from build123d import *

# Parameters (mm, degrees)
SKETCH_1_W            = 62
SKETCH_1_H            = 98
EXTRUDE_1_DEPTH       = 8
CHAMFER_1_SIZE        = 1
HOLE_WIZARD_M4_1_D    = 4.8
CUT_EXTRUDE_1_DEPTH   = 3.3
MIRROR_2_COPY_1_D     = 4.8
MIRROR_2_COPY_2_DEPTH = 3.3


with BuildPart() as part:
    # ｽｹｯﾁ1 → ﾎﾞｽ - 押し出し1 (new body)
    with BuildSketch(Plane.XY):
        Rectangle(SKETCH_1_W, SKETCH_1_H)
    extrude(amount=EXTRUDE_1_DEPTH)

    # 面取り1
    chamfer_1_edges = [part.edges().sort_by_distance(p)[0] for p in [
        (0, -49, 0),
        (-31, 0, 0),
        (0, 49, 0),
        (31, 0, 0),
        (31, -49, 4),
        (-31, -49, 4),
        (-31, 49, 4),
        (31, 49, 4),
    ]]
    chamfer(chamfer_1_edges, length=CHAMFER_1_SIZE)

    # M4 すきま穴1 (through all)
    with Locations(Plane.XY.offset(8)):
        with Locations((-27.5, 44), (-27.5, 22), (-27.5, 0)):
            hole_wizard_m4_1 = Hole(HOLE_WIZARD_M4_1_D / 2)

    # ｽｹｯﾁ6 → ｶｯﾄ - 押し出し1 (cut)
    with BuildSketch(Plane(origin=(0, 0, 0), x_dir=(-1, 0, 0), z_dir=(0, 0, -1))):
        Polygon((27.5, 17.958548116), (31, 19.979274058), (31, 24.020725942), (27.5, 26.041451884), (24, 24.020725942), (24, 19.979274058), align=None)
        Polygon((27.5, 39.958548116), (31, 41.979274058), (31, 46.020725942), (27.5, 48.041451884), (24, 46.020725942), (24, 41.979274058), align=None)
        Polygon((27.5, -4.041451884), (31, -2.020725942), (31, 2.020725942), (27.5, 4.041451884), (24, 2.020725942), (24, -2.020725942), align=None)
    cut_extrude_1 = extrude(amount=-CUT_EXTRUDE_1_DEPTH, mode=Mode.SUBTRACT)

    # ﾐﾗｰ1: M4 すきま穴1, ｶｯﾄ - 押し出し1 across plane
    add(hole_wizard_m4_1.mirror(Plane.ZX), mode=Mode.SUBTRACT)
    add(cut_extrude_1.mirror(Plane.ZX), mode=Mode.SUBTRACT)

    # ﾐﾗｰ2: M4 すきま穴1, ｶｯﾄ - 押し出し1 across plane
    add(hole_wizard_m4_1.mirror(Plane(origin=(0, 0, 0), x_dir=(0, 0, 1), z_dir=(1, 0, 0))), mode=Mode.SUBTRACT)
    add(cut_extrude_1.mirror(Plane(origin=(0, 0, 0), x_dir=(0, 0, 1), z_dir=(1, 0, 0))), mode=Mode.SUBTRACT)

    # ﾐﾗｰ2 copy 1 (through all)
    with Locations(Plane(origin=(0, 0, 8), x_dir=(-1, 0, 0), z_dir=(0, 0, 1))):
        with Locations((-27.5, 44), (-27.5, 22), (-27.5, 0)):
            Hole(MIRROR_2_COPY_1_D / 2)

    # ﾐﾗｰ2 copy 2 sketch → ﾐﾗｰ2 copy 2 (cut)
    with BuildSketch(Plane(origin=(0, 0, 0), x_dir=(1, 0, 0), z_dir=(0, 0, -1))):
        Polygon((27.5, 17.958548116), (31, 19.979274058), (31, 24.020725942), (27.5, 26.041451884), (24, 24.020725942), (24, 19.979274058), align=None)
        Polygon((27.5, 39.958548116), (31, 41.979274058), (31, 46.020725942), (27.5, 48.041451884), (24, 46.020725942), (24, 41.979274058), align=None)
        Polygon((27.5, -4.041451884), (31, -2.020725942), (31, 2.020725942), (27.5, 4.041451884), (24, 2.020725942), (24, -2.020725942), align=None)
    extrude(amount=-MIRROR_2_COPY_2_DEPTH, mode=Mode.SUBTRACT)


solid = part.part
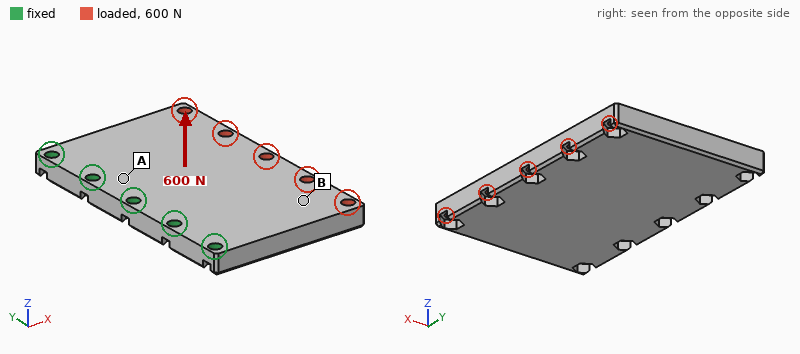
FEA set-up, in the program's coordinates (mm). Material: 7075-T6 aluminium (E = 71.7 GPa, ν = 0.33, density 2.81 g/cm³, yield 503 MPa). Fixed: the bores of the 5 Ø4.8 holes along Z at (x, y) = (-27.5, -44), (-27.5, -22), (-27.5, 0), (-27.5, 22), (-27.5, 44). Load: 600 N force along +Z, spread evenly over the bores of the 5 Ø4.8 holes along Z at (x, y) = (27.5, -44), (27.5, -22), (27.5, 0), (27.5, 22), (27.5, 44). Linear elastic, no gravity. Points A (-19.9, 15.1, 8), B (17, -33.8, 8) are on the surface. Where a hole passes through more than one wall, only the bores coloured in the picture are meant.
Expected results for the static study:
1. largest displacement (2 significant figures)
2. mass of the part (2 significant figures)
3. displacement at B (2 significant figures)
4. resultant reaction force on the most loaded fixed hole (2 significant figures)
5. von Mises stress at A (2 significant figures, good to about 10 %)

0.19 mm
130 g
0.13 mm
200 N
24 MPa
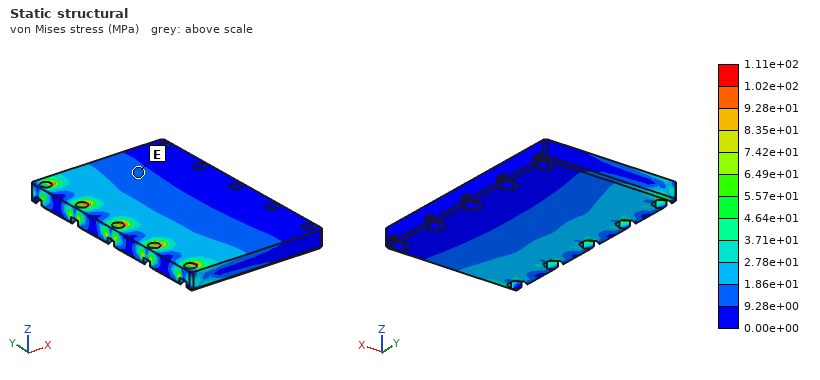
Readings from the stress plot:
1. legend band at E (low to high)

9.28e+00 to 1.86e+01 MPa
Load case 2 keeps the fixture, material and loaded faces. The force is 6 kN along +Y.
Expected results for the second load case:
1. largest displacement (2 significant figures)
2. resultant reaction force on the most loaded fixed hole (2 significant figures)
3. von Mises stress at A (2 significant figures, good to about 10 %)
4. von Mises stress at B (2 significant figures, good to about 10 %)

79 µm
3.2 kN
28 MPa
21 MPa
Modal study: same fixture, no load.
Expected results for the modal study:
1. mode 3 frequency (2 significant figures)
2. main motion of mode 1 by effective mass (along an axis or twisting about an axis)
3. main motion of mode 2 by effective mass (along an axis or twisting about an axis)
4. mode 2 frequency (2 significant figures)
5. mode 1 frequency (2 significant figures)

6300 Hz
along Z
twisting about X
2900 Hz
1500 Hz
